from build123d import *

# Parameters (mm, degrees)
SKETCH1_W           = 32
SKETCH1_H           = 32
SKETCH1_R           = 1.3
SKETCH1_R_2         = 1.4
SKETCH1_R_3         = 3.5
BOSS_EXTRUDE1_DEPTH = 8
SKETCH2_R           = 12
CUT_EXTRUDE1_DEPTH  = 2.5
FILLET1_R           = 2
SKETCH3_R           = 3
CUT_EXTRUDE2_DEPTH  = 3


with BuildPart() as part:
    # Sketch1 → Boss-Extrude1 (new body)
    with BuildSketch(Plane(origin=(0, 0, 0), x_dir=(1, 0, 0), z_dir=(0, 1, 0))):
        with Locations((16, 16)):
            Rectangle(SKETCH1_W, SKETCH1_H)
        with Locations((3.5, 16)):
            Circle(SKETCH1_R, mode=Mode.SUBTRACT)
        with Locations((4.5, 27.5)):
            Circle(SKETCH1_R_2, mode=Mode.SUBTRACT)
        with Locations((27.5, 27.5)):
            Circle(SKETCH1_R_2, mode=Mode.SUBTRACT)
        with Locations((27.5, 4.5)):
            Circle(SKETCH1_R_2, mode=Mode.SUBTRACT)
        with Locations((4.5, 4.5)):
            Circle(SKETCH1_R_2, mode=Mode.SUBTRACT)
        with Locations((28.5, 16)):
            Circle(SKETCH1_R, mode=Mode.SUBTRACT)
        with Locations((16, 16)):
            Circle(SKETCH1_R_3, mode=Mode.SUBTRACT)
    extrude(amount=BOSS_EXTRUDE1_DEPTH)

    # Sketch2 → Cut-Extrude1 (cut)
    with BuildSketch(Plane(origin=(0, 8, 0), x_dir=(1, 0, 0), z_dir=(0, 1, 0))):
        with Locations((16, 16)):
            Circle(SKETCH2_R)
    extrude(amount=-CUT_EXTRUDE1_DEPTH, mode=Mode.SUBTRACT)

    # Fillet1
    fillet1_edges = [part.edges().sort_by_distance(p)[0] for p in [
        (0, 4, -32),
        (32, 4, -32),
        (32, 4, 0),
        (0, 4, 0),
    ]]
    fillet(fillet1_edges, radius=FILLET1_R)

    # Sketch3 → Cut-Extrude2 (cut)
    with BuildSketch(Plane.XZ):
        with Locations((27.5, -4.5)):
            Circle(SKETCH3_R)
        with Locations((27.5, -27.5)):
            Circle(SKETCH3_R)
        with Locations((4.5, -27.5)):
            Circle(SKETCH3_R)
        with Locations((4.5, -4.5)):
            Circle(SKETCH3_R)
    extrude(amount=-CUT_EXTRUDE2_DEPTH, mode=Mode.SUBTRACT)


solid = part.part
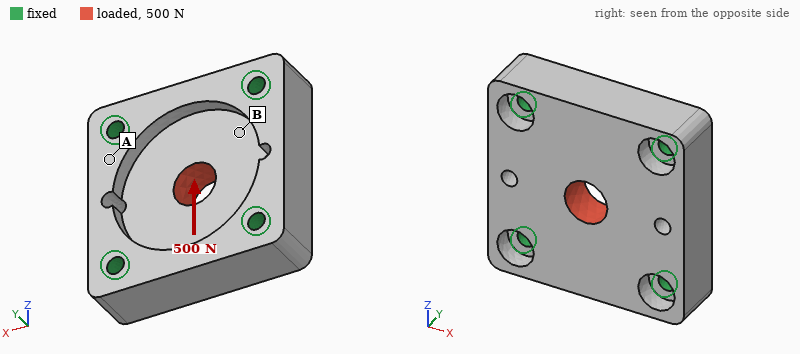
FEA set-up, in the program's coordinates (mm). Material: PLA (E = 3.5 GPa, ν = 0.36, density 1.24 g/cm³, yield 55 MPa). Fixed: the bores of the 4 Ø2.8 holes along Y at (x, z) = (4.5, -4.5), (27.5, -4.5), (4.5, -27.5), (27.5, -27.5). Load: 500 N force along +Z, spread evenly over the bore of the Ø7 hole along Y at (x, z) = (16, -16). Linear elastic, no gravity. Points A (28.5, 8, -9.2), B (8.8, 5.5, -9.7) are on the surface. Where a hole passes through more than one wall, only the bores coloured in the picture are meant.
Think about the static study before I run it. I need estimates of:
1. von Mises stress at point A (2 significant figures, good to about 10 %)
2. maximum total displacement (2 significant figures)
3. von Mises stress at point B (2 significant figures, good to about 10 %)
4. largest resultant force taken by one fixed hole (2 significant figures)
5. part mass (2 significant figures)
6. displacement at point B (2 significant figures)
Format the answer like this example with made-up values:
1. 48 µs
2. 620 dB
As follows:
1. 1.4 MPa
2. 20 µm
3. 4.2 MPa
4. 130 N
5. 7.8 g
6. 8.4 µm
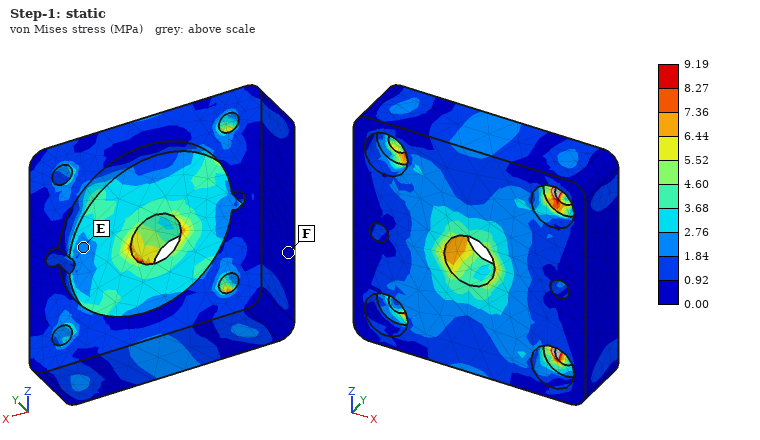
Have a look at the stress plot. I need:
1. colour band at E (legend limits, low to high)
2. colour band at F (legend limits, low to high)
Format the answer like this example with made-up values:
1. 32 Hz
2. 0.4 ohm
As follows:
1. 1.84 to 2.76 MPa
2. 0.00 to 0.92 MPa
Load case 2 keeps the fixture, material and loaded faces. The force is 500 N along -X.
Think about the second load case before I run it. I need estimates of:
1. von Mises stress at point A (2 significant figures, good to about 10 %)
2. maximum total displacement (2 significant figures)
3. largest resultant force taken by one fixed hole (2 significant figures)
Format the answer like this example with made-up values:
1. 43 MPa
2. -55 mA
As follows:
1. 1.1 MPa
2. 19 µm
3. 130 N
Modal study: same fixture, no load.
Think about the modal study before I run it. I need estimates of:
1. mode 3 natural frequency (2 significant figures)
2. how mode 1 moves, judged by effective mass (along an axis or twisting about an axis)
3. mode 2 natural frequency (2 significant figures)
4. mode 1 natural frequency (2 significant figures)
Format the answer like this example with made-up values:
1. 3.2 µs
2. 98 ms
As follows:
1. 14 kHz
2. along Y
3. 14 kHz
4. 11 kHz
